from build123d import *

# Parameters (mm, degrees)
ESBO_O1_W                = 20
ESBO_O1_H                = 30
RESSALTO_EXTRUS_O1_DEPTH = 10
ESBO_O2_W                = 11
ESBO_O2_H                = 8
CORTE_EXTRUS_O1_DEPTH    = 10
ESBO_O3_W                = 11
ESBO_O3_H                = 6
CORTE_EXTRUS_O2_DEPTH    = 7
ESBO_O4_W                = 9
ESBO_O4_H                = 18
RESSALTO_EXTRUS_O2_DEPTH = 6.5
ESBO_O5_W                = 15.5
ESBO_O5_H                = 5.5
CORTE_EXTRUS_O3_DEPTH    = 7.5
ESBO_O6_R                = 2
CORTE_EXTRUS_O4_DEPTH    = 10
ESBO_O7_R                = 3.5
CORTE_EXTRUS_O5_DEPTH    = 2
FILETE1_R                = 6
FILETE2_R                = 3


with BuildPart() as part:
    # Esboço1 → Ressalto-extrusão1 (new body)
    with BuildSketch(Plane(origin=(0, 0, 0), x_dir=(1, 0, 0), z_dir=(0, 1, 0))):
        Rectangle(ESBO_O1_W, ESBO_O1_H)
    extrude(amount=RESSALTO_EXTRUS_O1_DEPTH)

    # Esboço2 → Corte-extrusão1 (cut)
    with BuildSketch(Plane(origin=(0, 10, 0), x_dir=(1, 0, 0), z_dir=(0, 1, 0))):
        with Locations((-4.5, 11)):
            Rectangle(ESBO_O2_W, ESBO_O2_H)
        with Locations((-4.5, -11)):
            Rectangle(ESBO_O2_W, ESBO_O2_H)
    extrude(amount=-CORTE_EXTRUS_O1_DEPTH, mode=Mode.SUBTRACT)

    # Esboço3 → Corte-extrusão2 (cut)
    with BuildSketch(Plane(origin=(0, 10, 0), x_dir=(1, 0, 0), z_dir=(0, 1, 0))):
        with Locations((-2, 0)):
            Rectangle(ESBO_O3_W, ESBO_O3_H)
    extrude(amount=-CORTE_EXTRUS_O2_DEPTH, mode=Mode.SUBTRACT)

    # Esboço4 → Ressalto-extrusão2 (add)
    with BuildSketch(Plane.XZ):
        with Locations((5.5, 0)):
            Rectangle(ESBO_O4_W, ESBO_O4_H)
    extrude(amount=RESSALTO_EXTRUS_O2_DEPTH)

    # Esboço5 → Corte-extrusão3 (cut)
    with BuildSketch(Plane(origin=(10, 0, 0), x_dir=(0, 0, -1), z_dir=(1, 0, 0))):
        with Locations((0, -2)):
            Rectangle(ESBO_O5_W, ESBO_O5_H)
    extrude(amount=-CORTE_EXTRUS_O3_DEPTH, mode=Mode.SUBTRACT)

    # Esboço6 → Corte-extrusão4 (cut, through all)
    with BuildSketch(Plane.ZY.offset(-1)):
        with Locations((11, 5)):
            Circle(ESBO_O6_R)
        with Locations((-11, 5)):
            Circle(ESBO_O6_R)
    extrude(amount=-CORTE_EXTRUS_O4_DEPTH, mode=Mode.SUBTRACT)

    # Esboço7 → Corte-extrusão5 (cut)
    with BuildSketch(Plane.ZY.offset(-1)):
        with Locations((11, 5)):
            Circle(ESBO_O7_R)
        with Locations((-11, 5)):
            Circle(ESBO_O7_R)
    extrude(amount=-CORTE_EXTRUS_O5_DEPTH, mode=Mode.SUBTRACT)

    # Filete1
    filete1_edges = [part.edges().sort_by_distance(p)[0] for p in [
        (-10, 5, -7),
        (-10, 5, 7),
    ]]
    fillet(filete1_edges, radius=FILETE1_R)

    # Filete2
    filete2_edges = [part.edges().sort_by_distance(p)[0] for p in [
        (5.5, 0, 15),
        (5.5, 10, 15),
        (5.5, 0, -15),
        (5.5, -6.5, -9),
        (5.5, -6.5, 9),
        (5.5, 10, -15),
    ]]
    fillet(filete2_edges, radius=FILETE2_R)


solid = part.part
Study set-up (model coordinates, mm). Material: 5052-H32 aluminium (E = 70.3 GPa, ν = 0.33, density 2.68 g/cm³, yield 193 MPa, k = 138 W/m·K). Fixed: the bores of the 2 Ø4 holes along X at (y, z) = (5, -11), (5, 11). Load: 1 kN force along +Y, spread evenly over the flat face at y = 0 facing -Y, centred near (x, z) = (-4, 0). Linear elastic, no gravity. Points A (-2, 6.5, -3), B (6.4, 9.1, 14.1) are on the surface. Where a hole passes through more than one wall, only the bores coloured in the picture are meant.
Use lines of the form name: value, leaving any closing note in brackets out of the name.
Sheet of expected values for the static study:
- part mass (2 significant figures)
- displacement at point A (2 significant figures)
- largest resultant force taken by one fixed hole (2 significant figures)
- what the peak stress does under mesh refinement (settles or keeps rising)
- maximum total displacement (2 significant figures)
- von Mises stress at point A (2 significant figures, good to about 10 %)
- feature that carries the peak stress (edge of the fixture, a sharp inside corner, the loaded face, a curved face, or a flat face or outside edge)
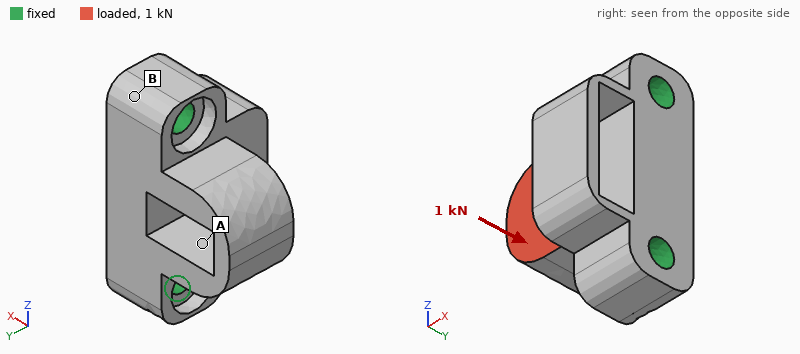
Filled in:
part mass: 9.7 g
displacement at point A: 14 µm
largest resultant force taken by one fixed hole: 500 N
what the peak stress does under mesh refinement: keeps rising
maximum total displacement: 30 µm
von Mises stress at point A: 19 MPa
feature that carries the peak stress: edge of the fixture
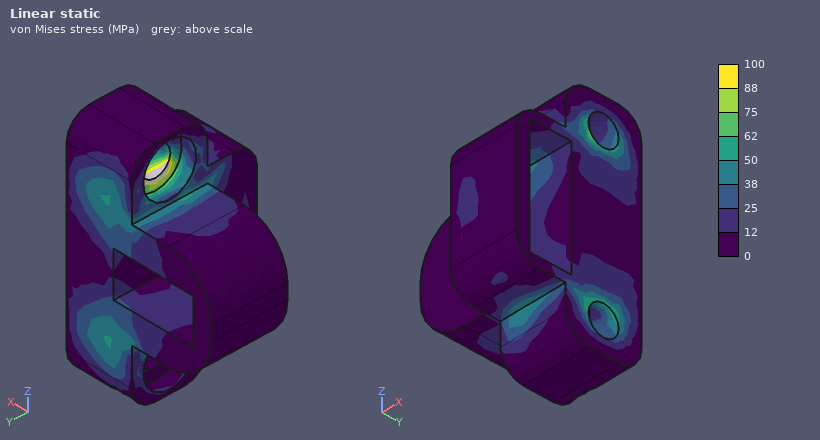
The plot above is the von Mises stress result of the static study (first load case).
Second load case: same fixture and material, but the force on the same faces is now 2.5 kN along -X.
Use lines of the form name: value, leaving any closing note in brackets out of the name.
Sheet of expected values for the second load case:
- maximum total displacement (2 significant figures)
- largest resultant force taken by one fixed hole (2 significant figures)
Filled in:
maximum total displacement: 44 µm
largest resultant force taken by one fixed hole: 1.3 kN
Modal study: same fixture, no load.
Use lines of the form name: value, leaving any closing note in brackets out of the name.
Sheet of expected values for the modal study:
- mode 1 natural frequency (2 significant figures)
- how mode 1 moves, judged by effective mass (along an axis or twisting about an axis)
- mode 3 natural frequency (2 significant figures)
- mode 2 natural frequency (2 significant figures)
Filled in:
mode 1 natural frequency: 19 kHz
how mode 1 moves, judged by effective mass: along Y
mode 3 natural frequency: 28 kHz
mode 2 natural frequency: 28 kHz
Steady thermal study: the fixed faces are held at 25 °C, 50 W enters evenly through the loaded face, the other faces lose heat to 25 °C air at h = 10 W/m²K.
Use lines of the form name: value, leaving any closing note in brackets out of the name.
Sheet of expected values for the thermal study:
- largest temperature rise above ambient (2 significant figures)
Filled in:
largest temperature rise above ambient: 49 K
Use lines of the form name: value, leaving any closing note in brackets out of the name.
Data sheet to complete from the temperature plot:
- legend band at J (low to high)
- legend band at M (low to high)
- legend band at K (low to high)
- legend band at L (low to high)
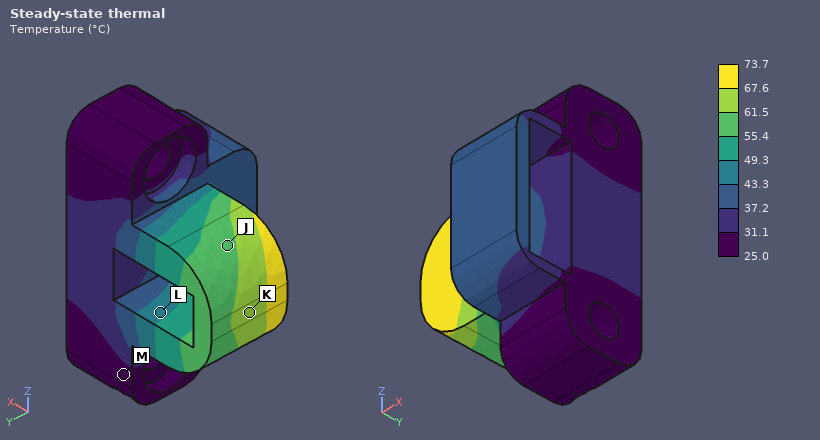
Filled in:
legend band at J: 55.4 to 61.5 °C
legend band at M: 25.0 to 31.1 °C
legend band at K: 61.5 to 67.6 °C
legend band at L: 43.3 to 49.3 °C
